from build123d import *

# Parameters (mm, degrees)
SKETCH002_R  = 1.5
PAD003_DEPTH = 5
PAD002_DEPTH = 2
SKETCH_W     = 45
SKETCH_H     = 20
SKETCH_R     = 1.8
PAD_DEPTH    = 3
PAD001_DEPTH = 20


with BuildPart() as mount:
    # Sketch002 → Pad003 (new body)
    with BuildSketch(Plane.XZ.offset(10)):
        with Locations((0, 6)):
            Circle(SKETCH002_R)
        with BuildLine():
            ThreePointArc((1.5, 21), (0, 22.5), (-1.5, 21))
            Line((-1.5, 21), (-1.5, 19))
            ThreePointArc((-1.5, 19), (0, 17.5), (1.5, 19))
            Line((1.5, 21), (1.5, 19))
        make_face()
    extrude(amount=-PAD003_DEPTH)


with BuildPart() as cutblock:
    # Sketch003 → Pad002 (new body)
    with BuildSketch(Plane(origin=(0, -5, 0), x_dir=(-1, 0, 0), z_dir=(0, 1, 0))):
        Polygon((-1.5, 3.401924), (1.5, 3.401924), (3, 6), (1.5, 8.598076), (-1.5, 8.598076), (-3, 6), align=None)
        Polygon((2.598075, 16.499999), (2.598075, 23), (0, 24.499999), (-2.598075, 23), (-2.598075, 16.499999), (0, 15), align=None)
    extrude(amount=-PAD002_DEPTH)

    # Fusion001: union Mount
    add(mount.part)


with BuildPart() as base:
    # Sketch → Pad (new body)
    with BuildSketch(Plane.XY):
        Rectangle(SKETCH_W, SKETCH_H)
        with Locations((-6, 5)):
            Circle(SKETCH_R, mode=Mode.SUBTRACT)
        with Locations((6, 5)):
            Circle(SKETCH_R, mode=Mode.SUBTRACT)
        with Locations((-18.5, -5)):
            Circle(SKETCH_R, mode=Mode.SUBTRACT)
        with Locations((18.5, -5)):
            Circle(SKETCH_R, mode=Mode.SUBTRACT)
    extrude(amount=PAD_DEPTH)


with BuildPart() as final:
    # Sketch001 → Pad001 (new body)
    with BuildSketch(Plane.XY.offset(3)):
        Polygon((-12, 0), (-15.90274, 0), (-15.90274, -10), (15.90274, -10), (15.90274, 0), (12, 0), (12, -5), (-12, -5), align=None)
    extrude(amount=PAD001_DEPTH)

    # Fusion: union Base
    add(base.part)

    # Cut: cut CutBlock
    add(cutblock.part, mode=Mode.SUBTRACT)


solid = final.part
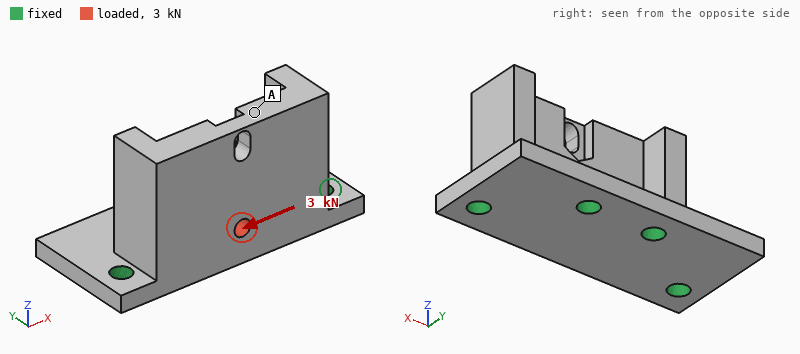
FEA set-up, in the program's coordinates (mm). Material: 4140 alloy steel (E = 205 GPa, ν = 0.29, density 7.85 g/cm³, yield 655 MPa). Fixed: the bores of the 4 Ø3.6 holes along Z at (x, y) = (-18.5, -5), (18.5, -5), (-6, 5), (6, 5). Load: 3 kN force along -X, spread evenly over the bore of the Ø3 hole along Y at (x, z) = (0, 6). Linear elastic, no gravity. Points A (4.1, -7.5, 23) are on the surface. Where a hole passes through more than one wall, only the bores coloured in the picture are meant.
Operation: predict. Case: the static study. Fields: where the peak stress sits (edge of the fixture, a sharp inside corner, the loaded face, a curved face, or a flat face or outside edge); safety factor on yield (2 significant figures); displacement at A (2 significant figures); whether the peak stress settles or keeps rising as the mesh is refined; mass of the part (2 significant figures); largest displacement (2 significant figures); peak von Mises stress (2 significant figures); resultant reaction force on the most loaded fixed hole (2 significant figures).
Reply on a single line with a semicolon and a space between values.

the loaded face; 3.4; 3.2 µm; settles; 50 g; 4.5 µm; 190 MPa; 1.2 kN
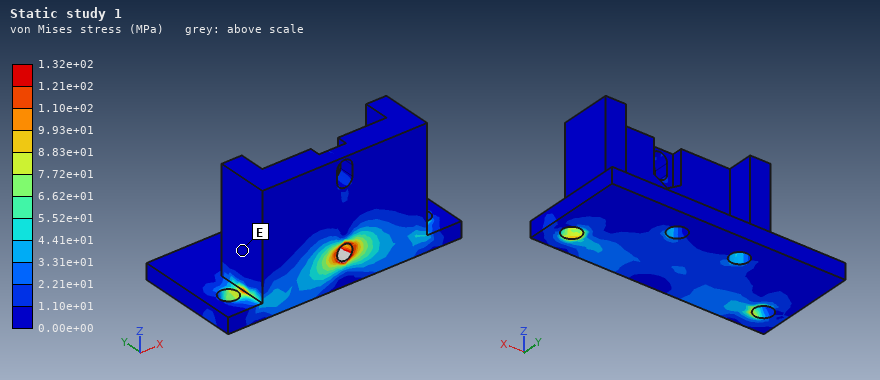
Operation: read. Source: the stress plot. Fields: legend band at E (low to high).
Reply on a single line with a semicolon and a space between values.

0.00e+00 to 1.10e+01 MPa
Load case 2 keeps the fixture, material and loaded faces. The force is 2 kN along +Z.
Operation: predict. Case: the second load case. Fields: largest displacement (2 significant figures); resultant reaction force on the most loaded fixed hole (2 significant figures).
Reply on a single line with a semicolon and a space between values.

25 µm; 1.2 kN
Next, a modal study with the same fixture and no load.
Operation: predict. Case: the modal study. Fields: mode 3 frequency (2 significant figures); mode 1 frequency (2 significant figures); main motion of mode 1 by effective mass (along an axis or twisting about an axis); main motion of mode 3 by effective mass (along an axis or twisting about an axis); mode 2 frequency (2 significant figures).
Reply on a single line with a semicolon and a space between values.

21 kHz; 6700 Hz; along Y; along X; 12 kHz
